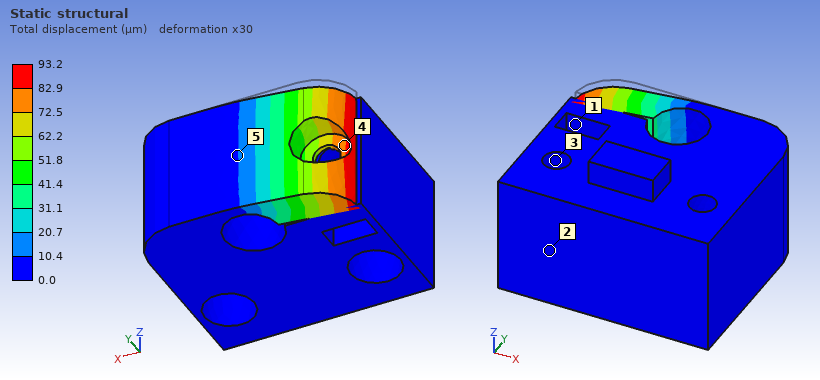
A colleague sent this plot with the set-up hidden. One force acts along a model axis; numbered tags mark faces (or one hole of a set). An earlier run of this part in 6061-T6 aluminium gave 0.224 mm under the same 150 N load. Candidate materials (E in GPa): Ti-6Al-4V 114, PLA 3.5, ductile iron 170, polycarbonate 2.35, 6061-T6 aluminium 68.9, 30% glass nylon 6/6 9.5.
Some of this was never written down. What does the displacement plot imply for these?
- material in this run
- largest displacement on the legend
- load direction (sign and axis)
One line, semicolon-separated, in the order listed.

ductile iron; 93.2 µm; -Y
